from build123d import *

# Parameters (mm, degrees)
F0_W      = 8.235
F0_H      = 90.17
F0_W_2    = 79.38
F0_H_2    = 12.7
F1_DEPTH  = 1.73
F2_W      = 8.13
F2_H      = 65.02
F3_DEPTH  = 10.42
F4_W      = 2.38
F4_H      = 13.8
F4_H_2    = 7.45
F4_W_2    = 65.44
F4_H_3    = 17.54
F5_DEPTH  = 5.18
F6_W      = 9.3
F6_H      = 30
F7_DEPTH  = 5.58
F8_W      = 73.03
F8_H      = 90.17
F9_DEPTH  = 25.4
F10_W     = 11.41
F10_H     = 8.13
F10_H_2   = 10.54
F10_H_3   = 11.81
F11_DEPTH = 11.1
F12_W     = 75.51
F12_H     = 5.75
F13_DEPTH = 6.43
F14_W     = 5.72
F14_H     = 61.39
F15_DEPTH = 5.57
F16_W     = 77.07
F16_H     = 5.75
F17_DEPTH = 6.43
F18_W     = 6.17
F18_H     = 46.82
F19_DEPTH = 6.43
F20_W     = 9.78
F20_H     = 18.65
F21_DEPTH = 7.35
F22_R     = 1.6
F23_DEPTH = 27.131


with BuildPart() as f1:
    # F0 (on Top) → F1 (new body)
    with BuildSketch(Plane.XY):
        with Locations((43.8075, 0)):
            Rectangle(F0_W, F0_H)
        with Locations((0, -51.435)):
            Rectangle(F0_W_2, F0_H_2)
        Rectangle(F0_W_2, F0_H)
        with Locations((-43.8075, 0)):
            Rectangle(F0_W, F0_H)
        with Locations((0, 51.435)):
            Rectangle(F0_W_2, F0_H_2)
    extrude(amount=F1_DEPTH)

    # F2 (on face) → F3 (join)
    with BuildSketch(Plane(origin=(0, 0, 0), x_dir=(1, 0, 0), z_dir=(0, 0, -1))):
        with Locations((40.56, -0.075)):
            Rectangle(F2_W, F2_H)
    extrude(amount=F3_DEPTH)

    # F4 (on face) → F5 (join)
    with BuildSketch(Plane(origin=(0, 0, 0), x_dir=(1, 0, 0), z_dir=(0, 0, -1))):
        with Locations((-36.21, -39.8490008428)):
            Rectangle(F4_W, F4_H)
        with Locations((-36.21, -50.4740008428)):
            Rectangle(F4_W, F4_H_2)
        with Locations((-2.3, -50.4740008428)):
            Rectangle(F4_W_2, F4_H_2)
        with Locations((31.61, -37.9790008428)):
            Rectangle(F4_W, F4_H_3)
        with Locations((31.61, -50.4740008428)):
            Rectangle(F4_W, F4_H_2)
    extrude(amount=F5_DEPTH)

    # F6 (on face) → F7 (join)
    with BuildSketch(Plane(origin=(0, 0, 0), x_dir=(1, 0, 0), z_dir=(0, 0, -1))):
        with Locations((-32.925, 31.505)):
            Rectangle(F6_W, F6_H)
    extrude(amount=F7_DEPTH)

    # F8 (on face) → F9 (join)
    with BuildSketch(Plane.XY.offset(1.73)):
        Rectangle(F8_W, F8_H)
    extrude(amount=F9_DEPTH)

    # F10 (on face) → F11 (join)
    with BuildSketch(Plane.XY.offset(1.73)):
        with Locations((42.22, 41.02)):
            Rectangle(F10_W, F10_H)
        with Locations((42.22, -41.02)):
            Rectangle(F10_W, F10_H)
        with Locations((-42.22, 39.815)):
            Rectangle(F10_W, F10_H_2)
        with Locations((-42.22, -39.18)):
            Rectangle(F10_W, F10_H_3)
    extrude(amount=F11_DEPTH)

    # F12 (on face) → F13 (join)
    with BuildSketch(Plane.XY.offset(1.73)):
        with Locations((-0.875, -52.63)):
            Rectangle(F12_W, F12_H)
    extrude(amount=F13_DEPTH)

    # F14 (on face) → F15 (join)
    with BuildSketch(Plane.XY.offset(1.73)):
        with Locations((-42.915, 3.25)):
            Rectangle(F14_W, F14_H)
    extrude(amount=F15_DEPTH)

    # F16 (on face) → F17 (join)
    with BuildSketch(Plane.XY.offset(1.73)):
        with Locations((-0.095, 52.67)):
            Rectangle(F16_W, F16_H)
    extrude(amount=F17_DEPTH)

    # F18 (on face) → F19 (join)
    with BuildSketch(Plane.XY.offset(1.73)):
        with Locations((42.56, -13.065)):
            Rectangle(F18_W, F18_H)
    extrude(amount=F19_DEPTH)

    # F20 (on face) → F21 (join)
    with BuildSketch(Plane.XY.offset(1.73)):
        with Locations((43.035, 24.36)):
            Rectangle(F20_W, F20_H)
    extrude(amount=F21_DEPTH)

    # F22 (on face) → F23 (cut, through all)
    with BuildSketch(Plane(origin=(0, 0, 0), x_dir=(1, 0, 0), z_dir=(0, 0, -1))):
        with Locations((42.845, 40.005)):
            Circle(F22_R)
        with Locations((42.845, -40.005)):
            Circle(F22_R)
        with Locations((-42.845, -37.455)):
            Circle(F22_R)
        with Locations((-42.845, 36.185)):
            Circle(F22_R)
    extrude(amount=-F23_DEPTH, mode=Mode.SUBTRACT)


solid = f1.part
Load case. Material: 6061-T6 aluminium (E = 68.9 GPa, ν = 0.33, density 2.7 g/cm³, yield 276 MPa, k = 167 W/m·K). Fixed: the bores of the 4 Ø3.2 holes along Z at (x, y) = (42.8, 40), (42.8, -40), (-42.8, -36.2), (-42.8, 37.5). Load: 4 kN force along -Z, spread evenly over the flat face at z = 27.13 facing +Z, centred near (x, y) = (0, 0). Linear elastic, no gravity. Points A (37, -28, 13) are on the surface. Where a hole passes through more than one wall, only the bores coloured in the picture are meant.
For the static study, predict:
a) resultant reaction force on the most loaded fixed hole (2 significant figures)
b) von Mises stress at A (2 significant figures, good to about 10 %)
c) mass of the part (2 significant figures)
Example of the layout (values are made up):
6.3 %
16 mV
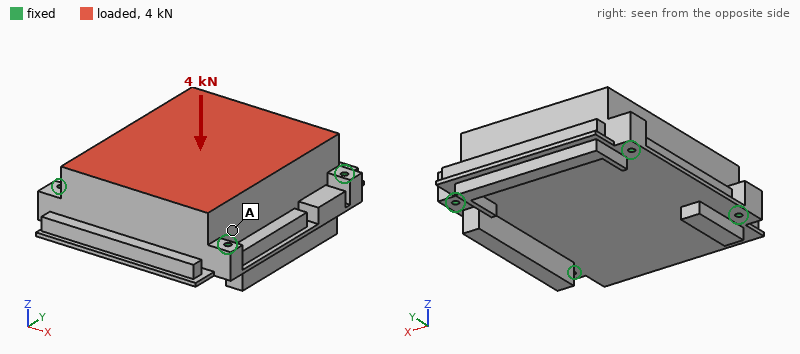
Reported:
1.1 kN
4.5 MPa
570 g
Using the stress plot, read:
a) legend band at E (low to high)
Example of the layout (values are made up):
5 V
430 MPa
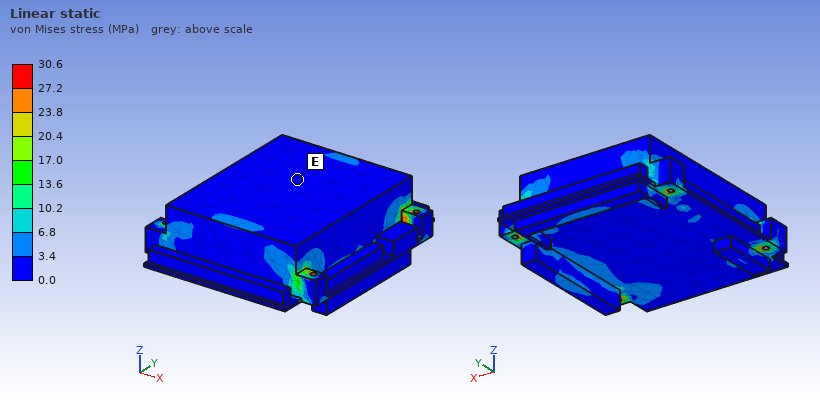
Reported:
0.0 to 3.4 MPa
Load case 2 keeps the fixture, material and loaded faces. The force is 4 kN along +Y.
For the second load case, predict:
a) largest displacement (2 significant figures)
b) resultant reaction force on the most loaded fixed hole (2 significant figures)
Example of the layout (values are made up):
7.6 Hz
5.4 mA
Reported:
8.2 µm
1.2 kN
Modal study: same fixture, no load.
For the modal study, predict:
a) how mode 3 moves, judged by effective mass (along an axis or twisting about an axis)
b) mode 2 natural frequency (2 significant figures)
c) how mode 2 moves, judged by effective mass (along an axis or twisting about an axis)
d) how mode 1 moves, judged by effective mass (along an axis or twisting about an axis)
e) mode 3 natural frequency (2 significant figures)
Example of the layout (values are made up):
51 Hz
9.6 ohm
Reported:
along Y
5200 Hz
along Z
along Z
6300 Hz
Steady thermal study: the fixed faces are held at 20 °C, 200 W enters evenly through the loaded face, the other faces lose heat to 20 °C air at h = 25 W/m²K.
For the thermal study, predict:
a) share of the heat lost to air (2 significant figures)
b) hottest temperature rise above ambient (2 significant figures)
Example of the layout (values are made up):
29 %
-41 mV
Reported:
7.9 %
29 K
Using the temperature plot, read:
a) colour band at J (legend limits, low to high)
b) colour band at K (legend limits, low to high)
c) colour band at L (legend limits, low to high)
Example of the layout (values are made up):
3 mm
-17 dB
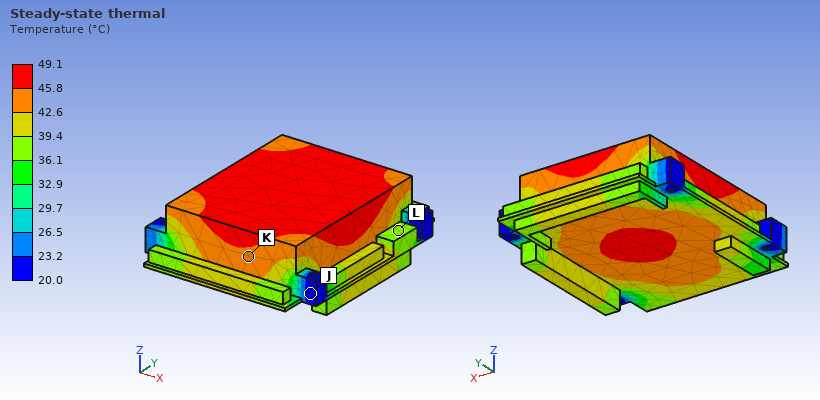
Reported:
20.0 to 23.2 °C
42.6 to 45.8 °C
36.1 to 39.4 °C
